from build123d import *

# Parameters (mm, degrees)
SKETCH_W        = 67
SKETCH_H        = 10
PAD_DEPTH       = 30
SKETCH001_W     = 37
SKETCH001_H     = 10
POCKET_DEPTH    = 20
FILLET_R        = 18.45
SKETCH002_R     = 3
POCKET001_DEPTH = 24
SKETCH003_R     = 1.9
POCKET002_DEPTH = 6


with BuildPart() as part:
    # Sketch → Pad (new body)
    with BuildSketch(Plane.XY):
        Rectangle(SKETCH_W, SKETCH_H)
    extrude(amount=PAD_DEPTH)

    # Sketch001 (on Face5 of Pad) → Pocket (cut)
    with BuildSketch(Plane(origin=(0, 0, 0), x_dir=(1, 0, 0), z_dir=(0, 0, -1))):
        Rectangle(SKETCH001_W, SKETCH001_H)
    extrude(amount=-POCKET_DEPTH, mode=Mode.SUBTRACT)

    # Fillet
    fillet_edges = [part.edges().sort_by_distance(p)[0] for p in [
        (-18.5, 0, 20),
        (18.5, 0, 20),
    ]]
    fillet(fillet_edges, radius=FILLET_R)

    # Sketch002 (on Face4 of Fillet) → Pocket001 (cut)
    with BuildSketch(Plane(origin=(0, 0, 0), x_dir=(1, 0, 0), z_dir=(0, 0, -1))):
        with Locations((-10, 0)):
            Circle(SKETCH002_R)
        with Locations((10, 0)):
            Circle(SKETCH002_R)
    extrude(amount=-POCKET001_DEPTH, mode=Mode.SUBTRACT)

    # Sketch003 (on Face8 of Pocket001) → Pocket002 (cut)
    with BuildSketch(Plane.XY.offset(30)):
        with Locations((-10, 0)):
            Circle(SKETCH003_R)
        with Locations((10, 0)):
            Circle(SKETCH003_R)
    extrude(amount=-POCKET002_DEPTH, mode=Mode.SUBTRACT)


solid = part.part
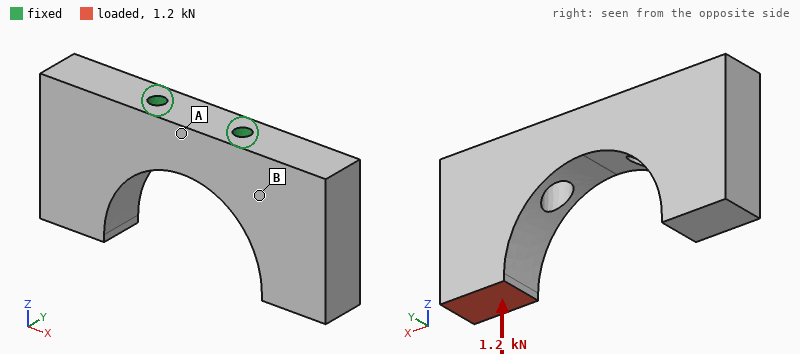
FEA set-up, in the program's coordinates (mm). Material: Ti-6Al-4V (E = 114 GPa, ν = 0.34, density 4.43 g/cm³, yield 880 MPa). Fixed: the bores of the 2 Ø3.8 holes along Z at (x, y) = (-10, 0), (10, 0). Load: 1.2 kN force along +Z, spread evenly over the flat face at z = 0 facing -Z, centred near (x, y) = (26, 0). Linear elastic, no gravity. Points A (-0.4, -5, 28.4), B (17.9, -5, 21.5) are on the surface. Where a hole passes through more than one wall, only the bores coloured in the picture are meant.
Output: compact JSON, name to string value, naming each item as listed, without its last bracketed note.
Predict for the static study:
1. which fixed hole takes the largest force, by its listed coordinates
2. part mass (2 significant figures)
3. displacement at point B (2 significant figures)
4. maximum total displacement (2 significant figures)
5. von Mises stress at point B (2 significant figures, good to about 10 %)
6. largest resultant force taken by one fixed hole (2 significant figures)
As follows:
{"which fixed hole takes the largest force, by its listed coordinates": "(10, 0)", "part mass": "60 g", "displacement at point B": "11 µm", "maximum total displacement": "51 µm", "von Mises stress at point B": "26 MPa", "largest resultant force taken by one fixed hole": "1.8 kN"}
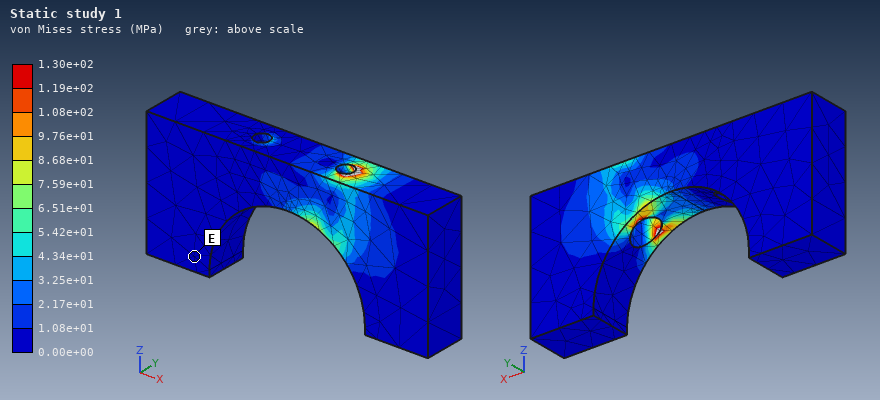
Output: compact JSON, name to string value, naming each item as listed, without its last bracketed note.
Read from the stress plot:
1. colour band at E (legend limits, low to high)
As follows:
{"colour band at E": "0.00e+00 to 1.08e+01 MPa"}
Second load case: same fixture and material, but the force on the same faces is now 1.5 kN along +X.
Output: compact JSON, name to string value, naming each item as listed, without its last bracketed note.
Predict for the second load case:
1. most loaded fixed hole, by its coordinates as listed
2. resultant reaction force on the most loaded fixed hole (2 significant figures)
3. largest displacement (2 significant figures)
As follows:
{"most loaded fixed hole, by its coordinates as listed": "(-10, 0)", "resultant reaction force on the most loaded fixed hole": "2.0 kN", "largest displacement": "0.12 mm"}
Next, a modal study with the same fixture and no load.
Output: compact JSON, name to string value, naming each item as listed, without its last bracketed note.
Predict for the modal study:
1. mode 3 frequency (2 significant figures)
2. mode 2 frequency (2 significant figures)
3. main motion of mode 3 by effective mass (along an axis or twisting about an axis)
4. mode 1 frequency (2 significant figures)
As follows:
{"mode 3 frequency": "5900 Hz", "mode 2 frequency": "5100 Hz", "main motion of mode 3 by effective mass": "along X", "mode 1 frequency": "5000 Hz"}
